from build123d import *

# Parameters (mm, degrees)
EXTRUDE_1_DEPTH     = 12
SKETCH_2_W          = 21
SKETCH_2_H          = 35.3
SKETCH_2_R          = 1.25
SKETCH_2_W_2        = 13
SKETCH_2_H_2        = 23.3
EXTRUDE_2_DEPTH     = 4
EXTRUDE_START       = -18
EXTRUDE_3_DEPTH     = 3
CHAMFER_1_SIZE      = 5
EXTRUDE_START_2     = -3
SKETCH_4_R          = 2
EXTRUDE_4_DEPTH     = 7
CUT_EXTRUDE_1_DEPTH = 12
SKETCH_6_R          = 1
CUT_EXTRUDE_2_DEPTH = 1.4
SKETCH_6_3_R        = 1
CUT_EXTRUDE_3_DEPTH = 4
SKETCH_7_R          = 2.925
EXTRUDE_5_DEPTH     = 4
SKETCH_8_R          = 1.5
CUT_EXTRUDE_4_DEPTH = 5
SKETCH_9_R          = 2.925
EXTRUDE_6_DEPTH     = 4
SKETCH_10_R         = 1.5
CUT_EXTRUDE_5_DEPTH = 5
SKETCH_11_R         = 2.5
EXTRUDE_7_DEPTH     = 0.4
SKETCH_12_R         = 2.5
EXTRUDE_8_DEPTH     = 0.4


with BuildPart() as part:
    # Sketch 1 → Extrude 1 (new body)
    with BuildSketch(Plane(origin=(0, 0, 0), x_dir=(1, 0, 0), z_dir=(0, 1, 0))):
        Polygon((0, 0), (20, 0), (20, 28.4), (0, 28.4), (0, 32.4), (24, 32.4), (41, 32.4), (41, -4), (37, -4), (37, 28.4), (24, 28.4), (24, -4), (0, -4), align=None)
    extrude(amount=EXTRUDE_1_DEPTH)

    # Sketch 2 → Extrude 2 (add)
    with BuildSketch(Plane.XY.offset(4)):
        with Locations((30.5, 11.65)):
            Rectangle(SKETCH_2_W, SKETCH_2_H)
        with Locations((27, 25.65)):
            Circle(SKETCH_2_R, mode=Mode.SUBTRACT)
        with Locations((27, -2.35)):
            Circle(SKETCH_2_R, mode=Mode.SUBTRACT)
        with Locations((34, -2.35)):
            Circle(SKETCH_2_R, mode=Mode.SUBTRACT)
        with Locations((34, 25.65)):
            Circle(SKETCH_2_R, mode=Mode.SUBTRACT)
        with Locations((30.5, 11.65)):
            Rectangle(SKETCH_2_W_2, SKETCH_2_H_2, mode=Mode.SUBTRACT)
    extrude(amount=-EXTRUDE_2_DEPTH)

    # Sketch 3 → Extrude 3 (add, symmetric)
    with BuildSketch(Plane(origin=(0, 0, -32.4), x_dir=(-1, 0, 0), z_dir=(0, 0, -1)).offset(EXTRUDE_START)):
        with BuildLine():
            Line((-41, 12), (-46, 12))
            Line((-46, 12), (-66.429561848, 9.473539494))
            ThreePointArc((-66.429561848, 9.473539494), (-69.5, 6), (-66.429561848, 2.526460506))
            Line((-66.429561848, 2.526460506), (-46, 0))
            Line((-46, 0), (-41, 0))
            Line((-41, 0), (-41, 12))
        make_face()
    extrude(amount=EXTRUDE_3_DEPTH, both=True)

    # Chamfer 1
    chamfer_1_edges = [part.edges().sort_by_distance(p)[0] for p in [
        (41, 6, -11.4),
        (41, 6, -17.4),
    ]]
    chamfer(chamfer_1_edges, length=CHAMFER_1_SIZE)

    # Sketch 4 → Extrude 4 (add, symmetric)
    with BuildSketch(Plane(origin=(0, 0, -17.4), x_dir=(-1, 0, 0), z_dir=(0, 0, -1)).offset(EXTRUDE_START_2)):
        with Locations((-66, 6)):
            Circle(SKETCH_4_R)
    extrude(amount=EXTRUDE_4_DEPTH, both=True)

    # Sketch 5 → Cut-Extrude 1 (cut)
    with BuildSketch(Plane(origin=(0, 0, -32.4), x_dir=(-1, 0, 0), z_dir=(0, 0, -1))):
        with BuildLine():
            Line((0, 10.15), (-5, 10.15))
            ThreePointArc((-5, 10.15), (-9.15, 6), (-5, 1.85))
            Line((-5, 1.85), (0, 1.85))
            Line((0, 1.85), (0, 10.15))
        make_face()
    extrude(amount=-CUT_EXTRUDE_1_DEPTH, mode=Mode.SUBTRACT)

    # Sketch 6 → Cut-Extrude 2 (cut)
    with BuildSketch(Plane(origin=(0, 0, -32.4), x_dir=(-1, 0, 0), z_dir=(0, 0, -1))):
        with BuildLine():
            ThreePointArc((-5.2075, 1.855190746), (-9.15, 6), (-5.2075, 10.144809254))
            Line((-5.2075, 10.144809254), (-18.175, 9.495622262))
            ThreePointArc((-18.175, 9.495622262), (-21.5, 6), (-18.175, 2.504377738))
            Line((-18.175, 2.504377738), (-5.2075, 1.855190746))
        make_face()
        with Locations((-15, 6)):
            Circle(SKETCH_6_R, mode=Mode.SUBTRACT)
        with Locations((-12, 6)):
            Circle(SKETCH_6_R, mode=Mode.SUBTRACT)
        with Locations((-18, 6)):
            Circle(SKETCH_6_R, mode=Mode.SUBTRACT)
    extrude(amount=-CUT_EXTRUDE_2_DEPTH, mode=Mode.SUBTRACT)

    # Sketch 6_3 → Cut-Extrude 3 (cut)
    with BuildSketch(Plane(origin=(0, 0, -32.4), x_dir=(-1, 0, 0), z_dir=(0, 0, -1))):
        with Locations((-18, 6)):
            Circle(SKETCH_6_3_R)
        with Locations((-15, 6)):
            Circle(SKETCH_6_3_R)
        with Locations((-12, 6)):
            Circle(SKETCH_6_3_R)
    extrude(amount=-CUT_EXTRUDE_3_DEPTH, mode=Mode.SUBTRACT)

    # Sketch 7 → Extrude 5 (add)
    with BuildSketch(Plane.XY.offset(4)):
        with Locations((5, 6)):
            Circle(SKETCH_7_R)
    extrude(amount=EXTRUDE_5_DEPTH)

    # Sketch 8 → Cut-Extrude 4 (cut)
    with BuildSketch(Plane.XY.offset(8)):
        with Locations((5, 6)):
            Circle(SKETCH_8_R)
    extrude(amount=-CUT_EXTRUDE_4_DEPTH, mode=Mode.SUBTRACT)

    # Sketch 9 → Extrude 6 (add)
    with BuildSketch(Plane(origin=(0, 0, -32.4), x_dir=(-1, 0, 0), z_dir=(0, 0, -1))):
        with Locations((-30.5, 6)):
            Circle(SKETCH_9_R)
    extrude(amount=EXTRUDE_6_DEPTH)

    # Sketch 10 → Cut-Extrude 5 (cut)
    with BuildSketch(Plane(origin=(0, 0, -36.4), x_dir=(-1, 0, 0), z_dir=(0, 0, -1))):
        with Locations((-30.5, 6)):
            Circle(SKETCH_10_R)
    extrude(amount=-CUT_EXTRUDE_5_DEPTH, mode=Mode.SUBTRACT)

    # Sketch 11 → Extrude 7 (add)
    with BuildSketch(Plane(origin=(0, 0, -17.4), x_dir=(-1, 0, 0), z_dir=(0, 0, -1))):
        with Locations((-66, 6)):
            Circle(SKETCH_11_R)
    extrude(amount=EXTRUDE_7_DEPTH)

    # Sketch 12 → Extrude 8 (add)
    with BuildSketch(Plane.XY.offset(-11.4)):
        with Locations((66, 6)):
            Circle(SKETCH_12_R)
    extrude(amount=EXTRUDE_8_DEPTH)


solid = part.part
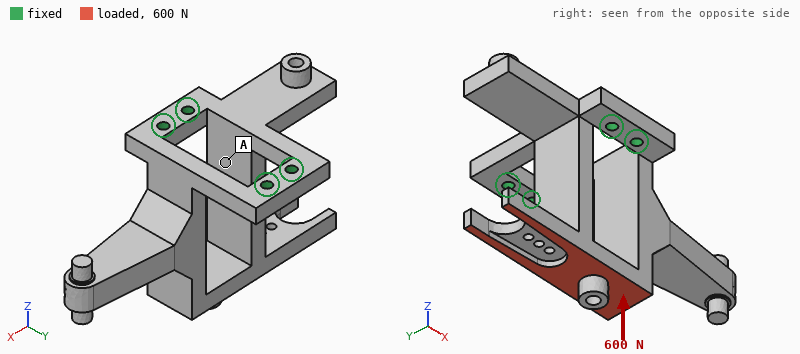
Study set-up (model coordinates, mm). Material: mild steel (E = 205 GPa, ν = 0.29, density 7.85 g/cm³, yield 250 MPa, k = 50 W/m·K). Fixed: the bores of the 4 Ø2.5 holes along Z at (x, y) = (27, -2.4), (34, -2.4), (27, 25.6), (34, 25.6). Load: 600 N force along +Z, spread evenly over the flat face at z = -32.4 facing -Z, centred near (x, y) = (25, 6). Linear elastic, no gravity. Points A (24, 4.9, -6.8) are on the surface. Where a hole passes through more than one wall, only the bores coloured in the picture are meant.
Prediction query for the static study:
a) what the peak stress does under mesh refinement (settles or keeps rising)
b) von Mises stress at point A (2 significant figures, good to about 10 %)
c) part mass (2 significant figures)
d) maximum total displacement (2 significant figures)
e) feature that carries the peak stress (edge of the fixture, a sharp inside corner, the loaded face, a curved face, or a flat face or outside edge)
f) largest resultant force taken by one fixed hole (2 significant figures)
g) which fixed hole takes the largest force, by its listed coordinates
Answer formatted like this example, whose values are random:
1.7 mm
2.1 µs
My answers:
keeps rising
11 MPa
71 g
57 µm
edge of the fixture
380 N
(27, -2.4)
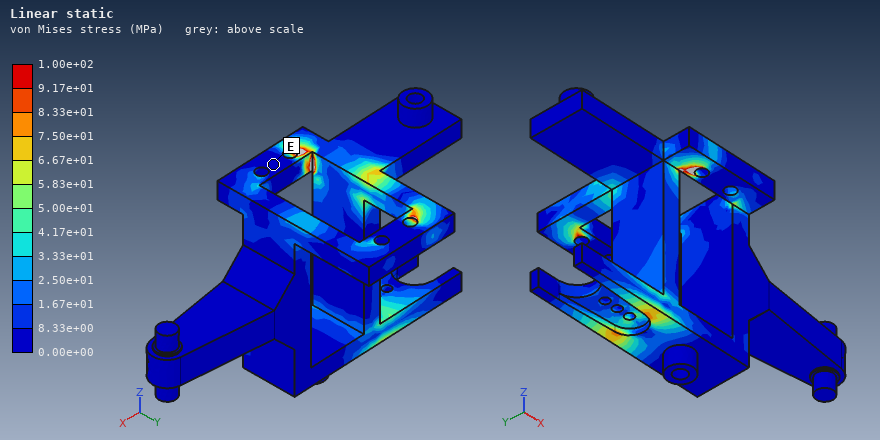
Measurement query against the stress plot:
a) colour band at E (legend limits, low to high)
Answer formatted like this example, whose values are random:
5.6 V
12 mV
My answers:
0.00e+00 to 8.33e+00 MPa
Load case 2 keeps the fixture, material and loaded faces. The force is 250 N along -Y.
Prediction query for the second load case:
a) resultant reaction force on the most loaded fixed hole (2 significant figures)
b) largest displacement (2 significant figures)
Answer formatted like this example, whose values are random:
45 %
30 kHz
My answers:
220 N
74 µm
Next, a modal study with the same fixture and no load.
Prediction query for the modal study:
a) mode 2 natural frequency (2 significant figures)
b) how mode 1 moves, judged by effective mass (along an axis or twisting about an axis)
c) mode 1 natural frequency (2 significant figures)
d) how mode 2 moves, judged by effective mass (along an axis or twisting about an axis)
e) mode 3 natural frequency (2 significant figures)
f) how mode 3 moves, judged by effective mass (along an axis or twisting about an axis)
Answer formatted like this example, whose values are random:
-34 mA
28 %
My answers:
2400 Hz
along X
1600 Hz
along Y
2800 Hz
twisting about Z
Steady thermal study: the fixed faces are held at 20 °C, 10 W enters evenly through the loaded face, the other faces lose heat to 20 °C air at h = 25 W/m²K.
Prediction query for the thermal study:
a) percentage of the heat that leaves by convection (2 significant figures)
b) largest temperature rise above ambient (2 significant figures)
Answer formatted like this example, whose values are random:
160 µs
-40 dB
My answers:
44 %
73 K
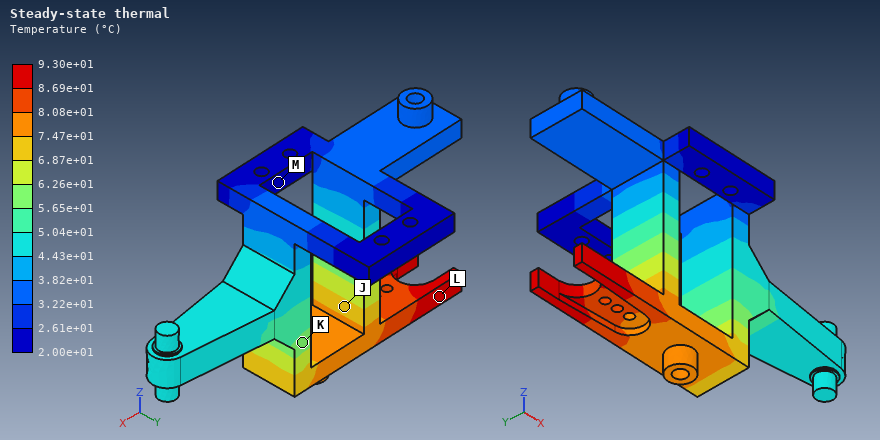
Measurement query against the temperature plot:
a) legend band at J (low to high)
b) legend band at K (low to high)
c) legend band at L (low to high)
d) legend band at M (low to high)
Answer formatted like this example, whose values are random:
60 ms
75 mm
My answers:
6.87e+01 to 7.47e+01 °C
5.65e+01 to 6.26e+01 °C
8.69e+01 to 9.30e+01 °C
2.00e+01 to 2.61e+01 °C
